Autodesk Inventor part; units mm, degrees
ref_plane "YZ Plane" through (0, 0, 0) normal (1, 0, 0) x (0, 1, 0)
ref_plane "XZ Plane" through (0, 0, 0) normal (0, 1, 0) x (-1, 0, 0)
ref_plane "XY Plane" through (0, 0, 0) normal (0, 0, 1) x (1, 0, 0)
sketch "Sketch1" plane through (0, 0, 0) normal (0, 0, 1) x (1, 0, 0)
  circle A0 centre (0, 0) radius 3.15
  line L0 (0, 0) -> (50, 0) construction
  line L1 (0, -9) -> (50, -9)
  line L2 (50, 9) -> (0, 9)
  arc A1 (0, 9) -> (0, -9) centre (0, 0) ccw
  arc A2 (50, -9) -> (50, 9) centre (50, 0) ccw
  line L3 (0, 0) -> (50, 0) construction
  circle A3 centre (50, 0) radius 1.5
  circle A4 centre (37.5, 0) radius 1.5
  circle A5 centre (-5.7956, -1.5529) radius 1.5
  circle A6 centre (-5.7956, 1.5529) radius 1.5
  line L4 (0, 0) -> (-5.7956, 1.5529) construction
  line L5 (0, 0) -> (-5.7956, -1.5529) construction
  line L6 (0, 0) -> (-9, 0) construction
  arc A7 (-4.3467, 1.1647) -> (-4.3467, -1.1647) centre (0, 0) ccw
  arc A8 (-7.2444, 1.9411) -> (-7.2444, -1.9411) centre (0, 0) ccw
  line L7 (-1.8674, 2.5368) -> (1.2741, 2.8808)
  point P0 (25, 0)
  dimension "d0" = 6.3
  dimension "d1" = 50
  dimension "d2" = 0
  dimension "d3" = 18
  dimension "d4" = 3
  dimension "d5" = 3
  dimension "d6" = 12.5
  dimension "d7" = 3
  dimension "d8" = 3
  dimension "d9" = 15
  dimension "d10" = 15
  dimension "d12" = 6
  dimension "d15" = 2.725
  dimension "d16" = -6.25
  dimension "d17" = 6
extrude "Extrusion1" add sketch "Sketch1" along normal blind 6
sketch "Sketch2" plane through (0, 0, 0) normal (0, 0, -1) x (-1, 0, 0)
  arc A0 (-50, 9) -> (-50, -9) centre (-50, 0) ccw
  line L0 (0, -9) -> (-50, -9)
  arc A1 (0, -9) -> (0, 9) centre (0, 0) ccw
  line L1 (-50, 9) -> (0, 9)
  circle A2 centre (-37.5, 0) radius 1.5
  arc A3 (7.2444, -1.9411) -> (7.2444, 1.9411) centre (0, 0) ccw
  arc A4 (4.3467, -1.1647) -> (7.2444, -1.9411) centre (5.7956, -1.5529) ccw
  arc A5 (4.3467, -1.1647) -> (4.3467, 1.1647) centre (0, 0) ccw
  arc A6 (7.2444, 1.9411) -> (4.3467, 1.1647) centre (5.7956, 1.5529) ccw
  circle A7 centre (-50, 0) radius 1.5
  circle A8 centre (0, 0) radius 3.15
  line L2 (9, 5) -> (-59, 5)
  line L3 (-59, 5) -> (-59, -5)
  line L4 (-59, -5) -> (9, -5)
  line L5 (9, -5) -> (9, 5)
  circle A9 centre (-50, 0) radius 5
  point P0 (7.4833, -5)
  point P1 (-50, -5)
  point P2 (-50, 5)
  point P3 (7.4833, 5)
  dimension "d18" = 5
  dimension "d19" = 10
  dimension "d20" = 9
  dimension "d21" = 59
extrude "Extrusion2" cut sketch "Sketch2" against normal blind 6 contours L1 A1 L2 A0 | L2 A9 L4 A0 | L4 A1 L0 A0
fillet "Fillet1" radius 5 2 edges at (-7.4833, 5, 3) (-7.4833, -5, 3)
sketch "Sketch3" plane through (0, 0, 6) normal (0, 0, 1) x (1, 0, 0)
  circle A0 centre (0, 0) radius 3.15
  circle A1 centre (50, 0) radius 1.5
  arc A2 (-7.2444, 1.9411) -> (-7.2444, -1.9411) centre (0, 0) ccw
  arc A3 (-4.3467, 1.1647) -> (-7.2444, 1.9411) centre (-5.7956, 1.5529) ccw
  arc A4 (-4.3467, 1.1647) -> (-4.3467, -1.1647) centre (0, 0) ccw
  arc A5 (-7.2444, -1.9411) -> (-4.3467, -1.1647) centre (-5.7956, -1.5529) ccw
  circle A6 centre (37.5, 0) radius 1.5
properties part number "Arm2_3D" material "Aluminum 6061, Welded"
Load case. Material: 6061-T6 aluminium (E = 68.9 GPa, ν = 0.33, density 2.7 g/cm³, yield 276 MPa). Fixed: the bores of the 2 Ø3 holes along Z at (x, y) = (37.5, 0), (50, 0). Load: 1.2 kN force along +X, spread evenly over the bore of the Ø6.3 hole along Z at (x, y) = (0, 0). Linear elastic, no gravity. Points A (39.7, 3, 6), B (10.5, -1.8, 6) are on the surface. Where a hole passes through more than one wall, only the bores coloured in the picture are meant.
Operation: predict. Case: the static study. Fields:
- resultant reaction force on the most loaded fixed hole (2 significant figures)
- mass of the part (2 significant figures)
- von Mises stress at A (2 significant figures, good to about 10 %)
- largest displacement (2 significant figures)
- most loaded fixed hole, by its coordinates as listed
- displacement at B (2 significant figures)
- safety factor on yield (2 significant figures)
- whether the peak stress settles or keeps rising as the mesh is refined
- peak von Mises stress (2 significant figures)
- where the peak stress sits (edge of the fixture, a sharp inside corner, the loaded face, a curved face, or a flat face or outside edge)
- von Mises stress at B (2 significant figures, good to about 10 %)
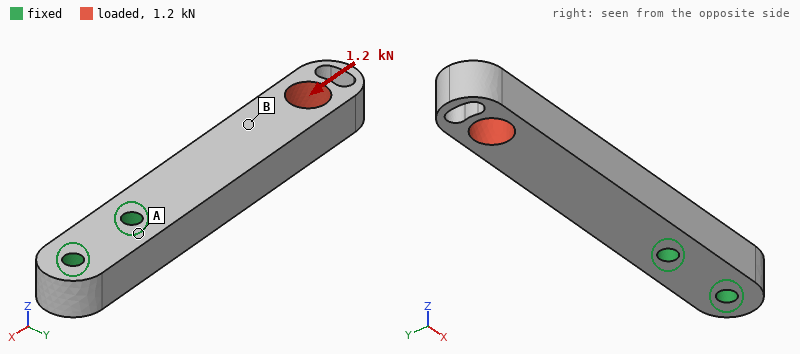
1.1 kN
9.0 g
7.2 MPa
18 µm
(37.5, 0)
8.0 µm
4.1
settles
68 MPa
the loaded face
19 MPa
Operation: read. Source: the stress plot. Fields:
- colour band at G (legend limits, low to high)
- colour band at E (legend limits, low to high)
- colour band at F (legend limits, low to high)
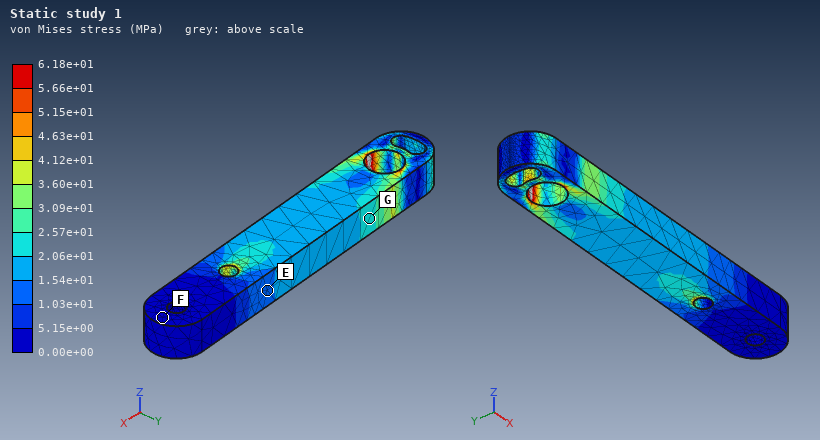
2.06e+01 to 2.57e+01 MPa
1.03e+01 to 1.54e+01 MPa
0.00e+00 to 5.15e+00 MPa
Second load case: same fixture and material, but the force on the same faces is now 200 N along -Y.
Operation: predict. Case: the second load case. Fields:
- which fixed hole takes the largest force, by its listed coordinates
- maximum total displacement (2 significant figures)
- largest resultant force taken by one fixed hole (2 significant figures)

(37.5, 0)
0.18 mm
510 N
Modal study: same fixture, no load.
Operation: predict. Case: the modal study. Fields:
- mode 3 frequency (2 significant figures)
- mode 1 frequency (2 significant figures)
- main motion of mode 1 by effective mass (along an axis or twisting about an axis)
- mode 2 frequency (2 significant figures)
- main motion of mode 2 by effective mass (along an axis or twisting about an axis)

14 kHz
2800 Hz
along Z
4000 Hz
along Y
